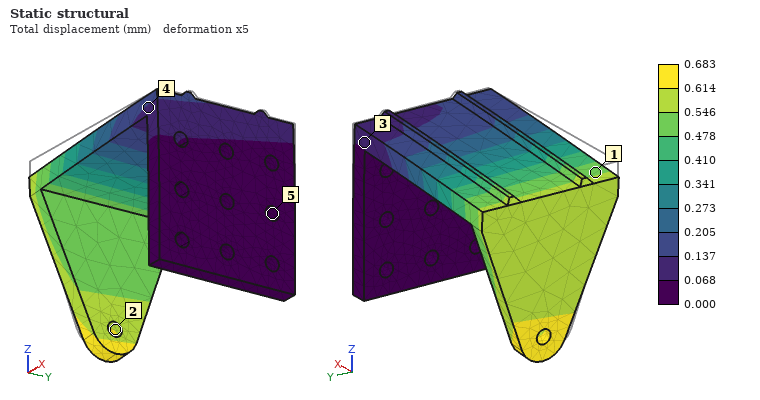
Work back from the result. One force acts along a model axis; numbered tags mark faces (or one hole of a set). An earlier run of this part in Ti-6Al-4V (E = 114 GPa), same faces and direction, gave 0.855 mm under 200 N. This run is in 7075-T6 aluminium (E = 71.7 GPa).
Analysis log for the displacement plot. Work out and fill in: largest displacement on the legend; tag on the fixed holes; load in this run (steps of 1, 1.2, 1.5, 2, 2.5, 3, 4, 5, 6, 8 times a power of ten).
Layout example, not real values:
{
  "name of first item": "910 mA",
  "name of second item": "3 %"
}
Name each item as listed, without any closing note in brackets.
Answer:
{
  "largest displacement on the legend": "0.683 mm",
  "tag on the fixed holes": "5",
  "load in this run": "100 N"
}
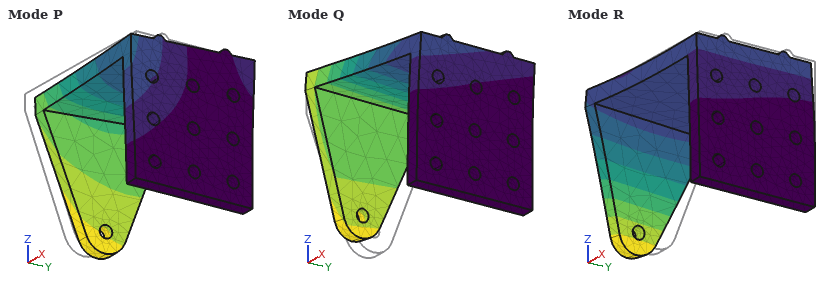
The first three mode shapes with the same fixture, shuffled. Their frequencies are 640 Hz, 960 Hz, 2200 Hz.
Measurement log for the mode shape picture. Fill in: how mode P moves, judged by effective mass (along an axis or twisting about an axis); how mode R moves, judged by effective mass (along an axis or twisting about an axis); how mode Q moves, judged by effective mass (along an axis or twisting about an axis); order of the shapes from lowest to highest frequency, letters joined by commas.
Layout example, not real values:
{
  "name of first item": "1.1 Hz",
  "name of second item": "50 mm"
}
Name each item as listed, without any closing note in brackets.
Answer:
{
  "how mode P moves, judged by effective mass": "along Y",
  "how mode R moves, judged by effective mass": "along X",
  "how mode Q moves, judged by effective mass": "along Z",
  "order of the shapes from lowest to highest frequency, letters joined by commas": "Q, P, R"
}
